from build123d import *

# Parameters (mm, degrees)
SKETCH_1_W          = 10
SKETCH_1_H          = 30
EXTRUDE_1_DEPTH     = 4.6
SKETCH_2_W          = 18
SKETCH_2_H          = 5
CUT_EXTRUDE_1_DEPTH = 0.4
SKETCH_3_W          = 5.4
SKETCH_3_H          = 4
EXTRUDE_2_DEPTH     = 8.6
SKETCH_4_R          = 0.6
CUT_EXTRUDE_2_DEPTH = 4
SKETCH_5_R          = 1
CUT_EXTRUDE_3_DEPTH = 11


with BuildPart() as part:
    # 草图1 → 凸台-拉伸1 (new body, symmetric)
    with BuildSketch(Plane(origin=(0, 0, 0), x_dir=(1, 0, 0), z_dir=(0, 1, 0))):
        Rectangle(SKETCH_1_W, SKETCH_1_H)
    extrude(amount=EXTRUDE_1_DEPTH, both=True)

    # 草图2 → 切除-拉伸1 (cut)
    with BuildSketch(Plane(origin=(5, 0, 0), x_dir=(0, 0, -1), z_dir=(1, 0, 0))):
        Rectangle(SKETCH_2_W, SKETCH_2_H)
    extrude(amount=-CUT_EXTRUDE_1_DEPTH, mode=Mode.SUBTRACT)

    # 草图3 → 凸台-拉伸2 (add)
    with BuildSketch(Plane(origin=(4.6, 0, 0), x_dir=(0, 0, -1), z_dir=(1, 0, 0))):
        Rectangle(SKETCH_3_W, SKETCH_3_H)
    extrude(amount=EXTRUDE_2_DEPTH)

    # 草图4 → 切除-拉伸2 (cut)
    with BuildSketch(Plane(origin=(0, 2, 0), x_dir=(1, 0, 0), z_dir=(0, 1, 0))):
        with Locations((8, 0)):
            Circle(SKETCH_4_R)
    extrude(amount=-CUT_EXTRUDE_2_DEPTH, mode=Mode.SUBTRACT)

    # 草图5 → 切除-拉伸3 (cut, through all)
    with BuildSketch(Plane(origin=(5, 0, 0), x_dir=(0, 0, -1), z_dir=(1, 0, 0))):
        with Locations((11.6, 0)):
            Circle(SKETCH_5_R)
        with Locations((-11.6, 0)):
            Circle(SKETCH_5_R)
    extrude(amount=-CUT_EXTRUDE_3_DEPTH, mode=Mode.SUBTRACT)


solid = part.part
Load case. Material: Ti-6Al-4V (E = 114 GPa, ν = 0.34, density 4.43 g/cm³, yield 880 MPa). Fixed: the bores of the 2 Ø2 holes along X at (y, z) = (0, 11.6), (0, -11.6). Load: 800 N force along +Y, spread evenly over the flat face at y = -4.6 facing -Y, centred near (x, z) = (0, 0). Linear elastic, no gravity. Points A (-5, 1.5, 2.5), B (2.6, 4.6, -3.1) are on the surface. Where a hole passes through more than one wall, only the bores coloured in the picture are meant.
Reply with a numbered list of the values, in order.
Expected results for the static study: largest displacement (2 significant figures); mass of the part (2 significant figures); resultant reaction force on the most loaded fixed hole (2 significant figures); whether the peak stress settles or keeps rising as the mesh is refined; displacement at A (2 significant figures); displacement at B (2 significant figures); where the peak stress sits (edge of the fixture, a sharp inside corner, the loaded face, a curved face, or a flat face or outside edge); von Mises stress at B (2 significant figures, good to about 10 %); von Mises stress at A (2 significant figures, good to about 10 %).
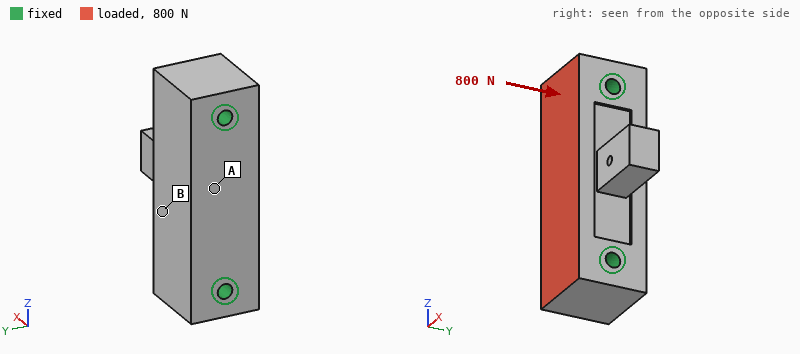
1. 1.5 µm
2. 13 g
3. 400 N
4. keeps rising
5. 1.1 µm
6. 1.1 µm
7. edge of the fixture
8. 7.4 MPa
9. 2.9 MPa
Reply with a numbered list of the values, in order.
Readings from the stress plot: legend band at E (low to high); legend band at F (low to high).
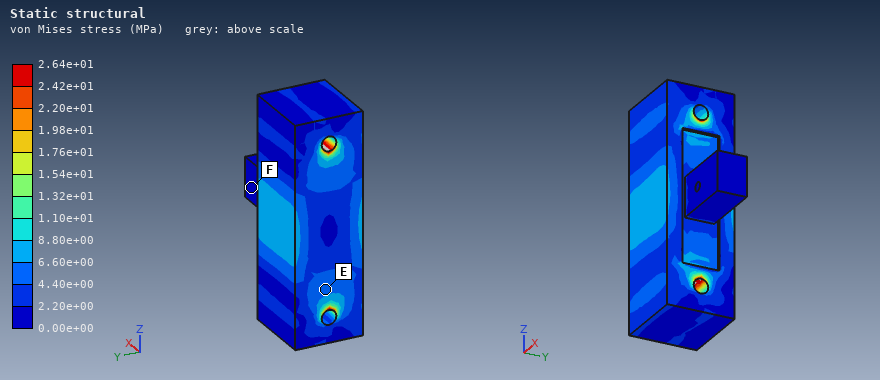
1. 4.40e+00 to 6.60e+00 MPa
2. 0.00e+00 to 2.20e+00 MPa
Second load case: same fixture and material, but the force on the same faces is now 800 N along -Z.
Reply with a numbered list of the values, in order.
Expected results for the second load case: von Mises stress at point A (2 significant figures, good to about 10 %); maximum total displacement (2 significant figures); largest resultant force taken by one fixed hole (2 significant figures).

1. 2.1 MPa
2. 0.73 µm
3. 420 N
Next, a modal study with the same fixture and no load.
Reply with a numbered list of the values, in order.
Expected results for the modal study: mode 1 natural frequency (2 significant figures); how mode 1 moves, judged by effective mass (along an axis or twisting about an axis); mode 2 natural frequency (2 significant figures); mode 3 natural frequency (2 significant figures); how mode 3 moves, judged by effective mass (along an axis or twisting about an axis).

1. 26 kHz
2. along Y
3. 37 kHz
4. 41 kHz
5. along Y
